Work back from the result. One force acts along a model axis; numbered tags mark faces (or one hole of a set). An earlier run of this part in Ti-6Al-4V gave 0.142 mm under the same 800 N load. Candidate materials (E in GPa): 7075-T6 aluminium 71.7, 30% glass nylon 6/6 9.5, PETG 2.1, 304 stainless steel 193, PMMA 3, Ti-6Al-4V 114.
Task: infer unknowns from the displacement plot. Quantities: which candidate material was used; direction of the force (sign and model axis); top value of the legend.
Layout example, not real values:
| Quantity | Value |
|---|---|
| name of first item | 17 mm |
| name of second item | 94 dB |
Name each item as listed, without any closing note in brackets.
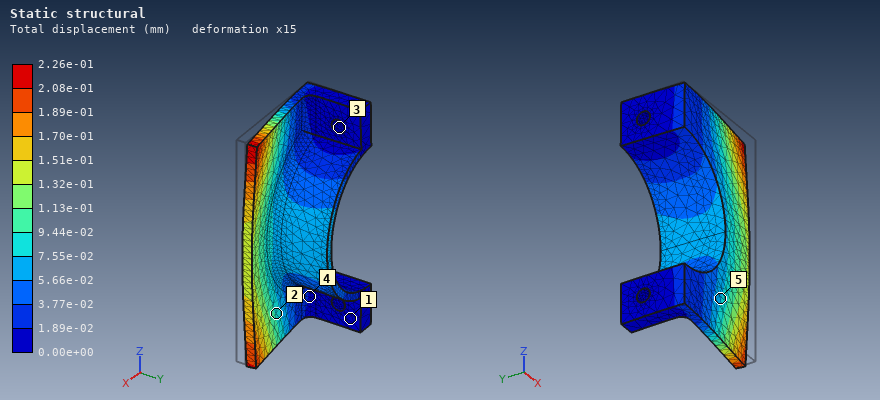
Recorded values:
| Quantity | Value |
|---|---|
| which candidate material was used | 7075-T6 aluminium |
| direction of the force | +Y |
| top value of the legend | 2.26e-01 mm |
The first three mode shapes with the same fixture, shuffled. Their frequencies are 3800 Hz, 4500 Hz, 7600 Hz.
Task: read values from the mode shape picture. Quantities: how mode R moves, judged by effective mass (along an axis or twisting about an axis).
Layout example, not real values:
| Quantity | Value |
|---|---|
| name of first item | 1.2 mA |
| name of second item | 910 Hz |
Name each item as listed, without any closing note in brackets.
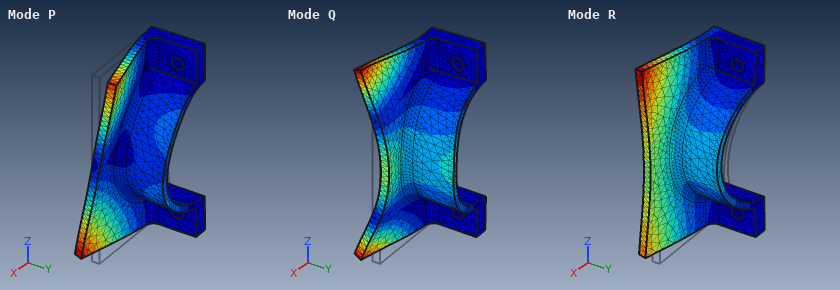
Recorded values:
| Quantity | Value |
|---|---|
| how mode R moves, judged by effective mass | along Y |
